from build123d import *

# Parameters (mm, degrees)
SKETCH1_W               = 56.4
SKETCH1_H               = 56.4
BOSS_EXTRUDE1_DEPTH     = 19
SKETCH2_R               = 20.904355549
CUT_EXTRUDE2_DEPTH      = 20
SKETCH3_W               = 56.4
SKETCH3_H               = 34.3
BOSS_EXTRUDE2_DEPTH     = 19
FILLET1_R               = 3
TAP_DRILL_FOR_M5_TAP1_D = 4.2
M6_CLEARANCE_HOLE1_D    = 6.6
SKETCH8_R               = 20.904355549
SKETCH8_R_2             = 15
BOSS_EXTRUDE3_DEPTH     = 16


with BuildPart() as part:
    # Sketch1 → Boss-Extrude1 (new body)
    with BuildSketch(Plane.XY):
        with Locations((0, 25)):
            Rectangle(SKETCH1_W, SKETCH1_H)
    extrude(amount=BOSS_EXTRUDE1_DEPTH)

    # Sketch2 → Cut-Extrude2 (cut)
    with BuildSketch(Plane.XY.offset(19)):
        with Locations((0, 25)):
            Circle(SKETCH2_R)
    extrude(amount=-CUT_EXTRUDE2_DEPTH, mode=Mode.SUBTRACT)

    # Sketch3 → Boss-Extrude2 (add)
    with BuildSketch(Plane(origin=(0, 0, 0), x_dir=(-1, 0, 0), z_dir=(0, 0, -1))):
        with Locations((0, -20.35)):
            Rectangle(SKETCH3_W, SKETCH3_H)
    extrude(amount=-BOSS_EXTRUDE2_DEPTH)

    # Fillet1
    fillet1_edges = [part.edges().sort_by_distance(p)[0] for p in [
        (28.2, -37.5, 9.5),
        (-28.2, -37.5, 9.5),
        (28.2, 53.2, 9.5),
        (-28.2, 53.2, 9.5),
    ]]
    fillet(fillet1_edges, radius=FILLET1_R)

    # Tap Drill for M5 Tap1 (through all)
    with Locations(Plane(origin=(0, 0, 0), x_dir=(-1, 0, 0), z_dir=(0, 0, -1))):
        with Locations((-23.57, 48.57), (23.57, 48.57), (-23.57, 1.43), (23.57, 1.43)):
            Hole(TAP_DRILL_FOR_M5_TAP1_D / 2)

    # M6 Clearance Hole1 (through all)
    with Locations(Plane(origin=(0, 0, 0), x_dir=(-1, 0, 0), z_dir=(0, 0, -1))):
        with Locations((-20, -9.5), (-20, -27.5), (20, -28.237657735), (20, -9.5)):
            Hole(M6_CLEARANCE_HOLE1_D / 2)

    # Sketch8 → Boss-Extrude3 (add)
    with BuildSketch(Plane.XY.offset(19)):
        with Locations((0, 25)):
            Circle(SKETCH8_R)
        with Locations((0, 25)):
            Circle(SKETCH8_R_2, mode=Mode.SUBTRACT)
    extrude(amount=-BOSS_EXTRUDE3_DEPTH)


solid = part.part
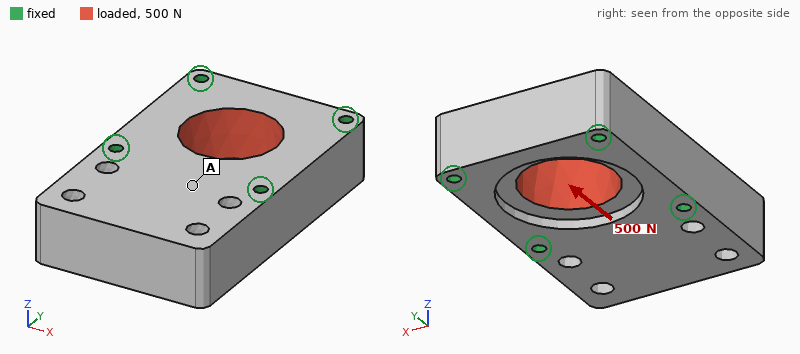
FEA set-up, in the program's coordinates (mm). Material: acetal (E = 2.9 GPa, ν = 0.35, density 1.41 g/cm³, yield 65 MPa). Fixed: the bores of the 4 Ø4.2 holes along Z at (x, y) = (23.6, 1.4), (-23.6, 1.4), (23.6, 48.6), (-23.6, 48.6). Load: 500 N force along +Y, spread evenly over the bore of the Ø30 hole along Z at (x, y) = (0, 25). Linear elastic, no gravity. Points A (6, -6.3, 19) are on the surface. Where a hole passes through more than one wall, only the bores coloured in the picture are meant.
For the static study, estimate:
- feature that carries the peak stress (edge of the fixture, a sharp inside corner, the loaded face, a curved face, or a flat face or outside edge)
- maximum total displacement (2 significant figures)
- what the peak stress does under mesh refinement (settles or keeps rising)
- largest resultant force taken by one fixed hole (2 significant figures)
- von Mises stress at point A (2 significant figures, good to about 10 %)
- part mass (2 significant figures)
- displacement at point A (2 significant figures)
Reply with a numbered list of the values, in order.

1. edge of the fixture
2. 9.3 µm
3. keeps rising
4. 140 N
5. 0.20 MPa
6. 110 g
7. 2.7 µm
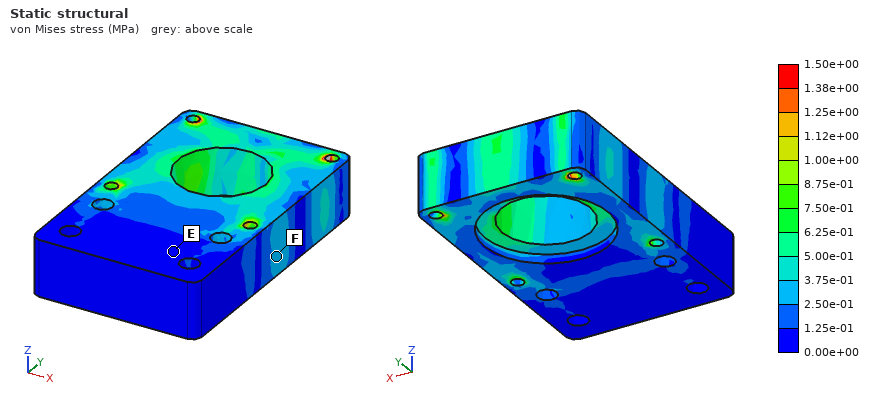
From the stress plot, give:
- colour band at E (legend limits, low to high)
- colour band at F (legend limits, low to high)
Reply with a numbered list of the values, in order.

1. 0.00e+00 to 1.25e-01 MPa
2. 2.50e-01 to 3.75e-01 MPa
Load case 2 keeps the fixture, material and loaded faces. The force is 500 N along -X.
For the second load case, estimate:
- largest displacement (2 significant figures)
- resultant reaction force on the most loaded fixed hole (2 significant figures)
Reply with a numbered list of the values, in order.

1. 8.4 µm
2. 140 N
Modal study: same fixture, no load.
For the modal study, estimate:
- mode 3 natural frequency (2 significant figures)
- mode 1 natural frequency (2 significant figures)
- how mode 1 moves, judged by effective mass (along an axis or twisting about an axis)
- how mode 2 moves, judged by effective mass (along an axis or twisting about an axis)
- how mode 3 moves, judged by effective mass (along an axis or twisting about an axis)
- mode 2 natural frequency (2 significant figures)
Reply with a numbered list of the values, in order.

1. 3900 Hz
2. 1800 Hz
3. along Z
4. twisting about Y
5. along X
6. 3700 Hz
